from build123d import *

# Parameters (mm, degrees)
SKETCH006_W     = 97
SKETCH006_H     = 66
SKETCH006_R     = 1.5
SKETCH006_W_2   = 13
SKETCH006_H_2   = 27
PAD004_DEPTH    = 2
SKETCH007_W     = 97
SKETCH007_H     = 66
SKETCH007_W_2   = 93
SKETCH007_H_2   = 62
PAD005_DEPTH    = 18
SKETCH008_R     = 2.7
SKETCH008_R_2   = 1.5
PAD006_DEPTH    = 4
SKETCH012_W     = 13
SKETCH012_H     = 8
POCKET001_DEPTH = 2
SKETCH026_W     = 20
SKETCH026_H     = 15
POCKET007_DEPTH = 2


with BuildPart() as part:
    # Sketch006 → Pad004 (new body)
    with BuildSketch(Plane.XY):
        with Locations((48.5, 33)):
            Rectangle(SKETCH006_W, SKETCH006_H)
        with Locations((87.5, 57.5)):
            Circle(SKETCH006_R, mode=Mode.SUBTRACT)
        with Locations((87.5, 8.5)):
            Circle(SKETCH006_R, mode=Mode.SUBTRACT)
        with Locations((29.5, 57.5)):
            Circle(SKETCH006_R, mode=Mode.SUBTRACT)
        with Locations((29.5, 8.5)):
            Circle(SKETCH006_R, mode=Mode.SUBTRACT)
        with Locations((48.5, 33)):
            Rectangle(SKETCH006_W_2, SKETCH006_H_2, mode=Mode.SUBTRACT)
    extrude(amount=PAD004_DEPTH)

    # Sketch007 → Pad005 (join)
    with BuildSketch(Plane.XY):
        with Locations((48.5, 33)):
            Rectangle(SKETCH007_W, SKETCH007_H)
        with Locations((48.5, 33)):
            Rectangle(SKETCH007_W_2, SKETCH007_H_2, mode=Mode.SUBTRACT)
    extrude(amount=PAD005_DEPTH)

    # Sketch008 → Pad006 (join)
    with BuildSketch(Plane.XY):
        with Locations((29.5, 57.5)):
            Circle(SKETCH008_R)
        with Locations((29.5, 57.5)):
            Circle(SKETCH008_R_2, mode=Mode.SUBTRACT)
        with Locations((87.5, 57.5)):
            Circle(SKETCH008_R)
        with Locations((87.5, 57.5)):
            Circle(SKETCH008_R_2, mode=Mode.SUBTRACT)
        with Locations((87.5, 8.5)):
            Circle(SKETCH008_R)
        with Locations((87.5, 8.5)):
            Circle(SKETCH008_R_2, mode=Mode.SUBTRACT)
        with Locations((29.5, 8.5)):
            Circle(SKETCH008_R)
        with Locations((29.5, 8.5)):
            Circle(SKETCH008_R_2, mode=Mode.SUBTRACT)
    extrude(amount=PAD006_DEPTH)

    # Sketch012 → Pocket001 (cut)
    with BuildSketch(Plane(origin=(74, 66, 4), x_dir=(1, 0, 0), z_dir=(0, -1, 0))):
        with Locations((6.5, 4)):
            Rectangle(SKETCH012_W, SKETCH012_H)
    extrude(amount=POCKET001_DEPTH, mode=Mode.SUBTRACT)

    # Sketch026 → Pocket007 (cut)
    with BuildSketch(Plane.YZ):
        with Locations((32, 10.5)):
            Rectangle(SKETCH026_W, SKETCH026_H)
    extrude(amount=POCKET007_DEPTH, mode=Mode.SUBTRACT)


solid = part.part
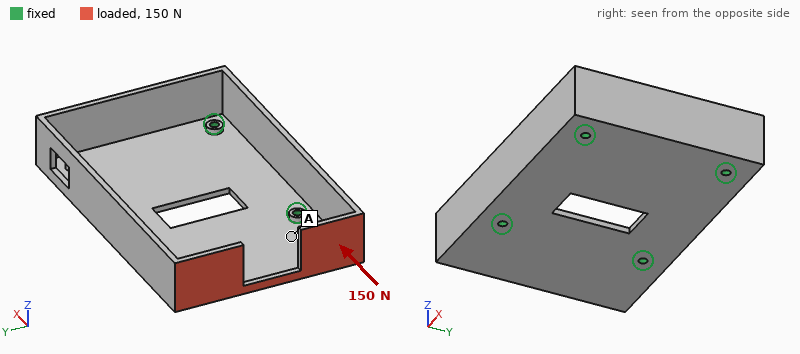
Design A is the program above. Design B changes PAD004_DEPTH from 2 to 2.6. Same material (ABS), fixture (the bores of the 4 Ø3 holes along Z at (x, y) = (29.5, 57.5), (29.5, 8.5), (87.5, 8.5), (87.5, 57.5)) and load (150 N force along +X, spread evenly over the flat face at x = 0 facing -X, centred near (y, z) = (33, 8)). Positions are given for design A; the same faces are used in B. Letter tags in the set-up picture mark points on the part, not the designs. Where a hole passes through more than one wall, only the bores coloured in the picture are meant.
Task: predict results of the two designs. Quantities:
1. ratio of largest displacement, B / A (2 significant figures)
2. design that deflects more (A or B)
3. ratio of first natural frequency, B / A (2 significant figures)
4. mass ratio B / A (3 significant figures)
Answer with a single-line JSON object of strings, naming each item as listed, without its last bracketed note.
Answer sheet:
{"ratio of largest displacement, B / A": "0.81", "design that deflects more": "A", "ratio of first natural frequency, B / A": "1.2", "mass ratio B / A": "1.15"}
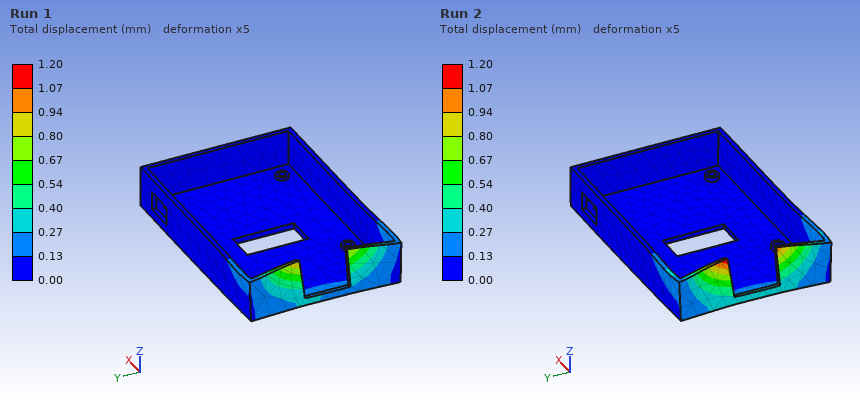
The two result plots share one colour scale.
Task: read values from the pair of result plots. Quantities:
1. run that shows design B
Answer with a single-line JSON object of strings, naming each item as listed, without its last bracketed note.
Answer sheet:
{"run that shows design B": "Run 1"}
